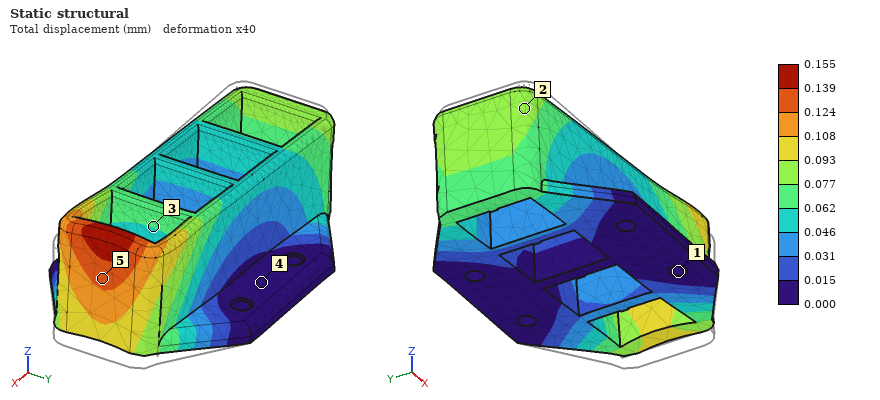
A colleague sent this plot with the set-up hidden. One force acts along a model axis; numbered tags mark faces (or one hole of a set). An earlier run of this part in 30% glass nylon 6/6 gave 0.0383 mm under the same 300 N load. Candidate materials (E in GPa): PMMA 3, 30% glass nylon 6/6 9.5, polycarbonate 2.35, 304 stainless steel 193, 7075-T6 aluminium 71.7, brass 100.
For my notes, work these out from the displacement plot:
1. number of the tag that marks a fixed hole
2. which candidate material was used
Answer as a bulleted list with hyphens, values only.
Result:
- 1
- polycarbonate
